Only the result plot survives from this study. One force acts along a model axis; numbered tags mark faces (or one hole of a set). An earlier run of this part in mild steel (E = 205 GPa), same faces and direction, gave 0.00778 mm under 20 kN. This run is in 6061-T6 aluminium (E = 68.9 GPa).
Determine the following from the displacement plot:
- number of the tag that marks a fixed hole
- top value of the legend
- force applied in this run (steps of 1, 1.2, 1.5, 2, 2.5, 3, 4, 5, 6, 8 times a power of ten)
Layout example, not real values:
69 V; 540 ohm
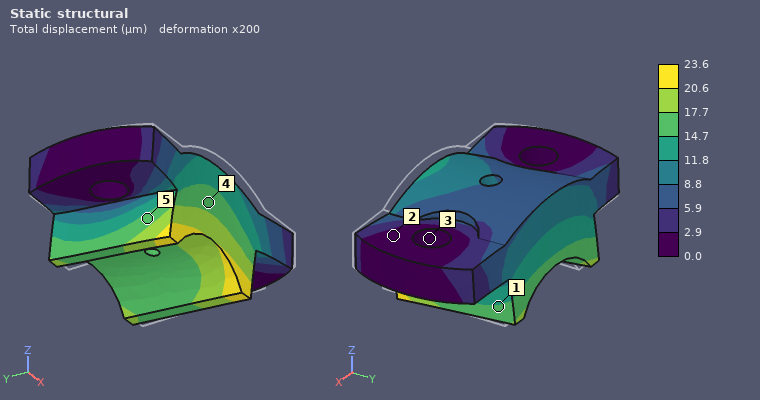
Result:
3; 23.6 µm; 20 kN
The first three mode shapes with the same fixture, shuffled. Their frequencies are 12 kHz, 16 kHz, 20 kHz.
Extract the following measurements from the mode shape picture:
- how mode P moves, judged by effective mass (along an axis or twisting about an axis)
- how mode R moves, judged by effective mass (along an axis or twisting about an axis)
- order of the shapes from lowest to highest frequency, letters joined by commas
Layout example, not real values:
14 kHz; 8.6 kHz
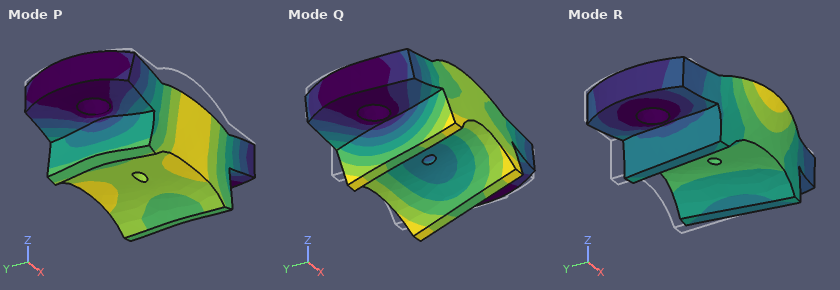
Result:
along Z; along Y; Q, P, R
